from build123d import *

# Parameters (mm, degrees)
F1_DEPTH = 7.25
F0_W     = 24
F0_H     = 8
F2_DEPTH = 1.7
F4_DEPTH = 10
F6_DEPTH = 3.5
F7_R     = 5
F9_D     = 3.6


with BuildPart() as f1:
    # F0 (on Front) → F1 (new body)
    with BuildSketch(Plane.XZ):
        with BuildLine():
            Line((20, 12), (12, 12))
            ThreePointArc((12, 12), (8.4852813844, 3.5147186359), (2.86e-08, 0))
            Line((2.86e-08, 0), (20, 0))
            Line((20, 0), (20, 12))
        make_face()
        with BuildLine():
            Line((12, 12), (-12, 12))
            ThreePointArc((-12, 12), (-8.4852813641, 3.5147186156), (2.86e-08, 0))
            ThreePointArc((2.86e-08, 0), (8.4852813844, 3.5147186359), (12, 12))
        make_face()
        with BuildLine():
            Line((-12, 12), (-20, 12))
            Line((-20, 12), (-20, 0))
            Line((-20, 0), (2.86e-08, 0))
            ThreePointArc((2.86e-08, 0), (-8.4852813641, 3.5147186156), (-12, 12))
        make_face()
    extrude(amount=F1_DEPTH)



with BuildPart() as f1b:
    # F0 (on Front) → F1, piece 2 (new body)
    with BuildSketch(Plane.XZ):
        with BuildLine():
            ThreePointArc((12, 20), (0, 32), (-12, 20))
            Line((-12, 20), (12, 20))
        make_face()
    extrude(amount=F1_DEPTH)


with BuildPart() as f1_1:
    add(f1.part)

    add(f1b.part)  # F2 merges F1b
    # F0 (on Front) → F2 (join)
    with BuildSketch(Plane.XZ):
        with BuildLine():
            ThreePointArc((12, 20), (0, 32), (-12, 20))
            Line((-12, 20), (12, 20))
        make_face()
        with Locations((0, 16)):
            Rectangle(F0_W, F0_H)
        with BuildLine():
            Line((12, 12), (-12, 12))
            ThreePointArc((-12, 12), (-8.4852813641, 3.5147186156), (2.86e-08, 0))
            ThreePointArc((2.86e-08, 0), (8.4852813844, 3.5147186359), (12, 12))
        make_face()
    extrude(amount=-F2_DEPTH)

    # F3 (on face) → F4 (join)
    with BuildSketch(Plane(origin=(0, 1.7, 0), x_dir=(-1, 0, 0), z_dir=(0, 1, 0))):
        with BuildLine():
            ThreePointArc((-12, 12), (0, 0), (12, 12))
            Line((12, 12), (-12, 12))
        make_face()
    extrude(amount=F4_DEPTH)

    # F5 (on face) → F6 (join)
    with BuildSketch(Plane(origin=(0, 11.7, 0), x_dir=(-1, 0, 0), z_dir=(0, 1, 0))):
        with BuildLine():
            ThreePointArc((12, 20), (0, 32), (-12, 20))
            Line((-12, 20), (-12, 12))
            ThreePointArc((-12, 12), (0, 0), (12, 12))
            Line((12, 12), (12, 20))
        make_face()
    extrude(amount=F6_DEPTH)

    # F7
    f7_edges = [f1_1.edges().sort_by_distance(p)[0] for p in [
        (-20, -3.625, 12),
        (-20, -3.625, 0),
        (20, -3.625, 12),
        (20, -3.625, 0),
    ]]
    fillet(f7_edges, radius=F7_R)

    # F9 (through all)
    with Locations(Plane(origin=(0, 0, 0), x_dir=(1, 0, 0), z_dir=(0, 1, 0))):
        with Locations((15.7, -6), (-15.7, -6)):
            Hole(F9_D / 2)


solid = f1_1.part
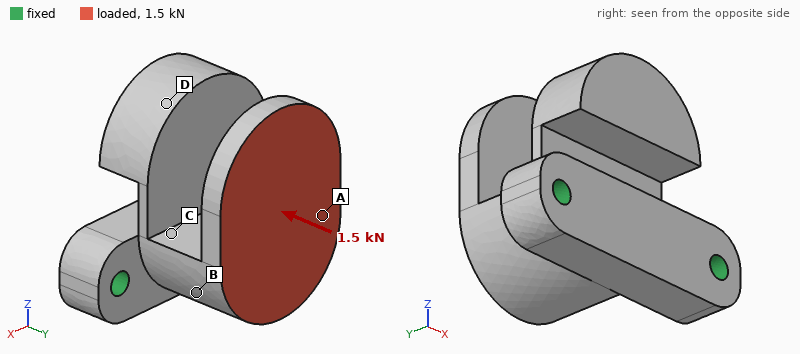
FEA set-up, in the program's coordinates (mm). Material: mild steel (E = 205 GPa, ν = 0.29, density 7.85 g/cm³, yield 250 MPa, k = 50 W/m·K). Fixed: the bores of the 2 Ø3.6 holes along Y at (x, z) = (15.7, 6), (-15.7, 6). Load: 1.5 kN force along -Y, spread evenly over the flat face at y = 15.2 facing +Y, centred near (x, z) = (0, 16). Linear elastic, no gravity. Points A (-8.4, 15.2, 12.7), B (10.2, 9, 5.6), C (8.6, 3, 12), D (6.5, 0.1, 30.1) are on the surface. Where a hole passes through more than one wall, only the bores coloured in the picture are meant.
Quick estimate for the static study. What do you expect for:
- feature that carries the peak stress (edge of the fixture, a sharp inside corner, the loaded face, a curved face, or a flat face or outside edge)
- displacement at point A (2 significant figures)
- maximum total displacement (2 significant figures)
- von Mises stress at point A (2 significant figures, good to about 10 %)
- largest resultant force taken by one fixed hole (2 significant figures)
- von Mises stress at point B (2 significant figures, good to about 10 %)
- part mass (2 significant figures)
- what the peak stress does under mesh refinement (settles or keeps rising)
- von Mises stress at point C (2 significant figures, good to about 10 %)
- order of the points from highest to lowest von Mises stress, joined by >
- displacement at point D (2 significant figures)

edge of the fixture
22 µm
99 µm
140 MPa
790 N
26 MPa
82 g
keeps rising
46 MPa
A > C > B > D
19 µm
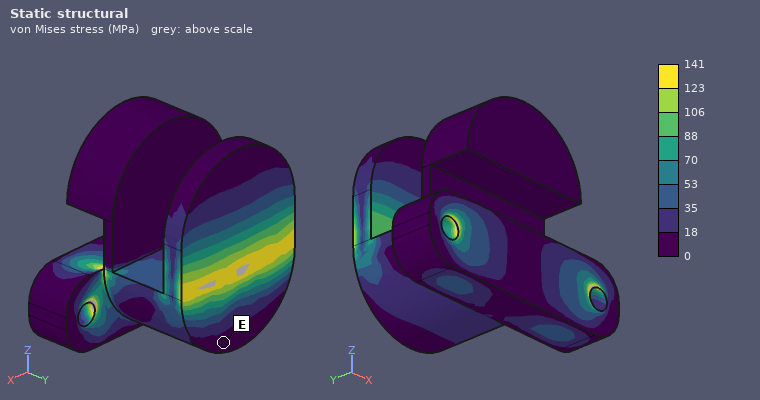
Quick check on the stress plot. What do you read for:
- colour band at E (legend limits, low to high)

0 to 18 MPa
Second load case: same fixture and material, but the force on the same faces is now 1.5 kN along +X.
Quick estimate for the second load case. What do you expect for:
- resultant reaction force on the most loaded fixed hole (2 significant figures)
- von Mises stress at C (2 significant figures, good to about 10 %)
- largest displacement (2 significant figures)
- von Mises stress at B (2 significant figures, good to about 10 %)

1.4 kN
46 MPa
20 µm
27 MPa
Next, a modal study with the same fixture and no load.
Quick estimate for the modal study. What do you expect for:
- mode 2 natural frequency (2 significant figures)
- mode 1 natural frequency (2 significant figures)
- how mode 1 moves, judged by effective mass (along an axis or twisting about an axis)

5300 Hz
1700 Hz
along Y
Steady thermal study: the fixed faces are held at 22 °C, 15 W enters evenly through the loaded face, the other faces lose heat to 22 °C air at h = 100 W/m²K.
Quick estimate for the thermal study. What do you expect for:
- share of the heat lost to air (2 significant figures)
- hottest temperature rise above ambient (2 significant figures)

36 %
44 K
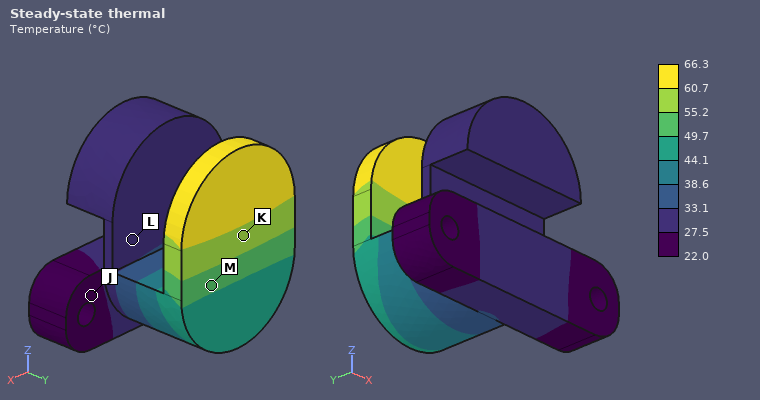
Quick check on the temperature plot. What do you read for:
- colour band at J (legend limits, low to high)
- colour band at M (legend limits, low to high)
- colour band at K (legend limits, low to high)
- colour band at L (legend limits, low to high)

22.0 to 27.5 °C
49.7 to 55.2 °C
55.2 to 60.7 °C
27.5 to 33.1 °C
